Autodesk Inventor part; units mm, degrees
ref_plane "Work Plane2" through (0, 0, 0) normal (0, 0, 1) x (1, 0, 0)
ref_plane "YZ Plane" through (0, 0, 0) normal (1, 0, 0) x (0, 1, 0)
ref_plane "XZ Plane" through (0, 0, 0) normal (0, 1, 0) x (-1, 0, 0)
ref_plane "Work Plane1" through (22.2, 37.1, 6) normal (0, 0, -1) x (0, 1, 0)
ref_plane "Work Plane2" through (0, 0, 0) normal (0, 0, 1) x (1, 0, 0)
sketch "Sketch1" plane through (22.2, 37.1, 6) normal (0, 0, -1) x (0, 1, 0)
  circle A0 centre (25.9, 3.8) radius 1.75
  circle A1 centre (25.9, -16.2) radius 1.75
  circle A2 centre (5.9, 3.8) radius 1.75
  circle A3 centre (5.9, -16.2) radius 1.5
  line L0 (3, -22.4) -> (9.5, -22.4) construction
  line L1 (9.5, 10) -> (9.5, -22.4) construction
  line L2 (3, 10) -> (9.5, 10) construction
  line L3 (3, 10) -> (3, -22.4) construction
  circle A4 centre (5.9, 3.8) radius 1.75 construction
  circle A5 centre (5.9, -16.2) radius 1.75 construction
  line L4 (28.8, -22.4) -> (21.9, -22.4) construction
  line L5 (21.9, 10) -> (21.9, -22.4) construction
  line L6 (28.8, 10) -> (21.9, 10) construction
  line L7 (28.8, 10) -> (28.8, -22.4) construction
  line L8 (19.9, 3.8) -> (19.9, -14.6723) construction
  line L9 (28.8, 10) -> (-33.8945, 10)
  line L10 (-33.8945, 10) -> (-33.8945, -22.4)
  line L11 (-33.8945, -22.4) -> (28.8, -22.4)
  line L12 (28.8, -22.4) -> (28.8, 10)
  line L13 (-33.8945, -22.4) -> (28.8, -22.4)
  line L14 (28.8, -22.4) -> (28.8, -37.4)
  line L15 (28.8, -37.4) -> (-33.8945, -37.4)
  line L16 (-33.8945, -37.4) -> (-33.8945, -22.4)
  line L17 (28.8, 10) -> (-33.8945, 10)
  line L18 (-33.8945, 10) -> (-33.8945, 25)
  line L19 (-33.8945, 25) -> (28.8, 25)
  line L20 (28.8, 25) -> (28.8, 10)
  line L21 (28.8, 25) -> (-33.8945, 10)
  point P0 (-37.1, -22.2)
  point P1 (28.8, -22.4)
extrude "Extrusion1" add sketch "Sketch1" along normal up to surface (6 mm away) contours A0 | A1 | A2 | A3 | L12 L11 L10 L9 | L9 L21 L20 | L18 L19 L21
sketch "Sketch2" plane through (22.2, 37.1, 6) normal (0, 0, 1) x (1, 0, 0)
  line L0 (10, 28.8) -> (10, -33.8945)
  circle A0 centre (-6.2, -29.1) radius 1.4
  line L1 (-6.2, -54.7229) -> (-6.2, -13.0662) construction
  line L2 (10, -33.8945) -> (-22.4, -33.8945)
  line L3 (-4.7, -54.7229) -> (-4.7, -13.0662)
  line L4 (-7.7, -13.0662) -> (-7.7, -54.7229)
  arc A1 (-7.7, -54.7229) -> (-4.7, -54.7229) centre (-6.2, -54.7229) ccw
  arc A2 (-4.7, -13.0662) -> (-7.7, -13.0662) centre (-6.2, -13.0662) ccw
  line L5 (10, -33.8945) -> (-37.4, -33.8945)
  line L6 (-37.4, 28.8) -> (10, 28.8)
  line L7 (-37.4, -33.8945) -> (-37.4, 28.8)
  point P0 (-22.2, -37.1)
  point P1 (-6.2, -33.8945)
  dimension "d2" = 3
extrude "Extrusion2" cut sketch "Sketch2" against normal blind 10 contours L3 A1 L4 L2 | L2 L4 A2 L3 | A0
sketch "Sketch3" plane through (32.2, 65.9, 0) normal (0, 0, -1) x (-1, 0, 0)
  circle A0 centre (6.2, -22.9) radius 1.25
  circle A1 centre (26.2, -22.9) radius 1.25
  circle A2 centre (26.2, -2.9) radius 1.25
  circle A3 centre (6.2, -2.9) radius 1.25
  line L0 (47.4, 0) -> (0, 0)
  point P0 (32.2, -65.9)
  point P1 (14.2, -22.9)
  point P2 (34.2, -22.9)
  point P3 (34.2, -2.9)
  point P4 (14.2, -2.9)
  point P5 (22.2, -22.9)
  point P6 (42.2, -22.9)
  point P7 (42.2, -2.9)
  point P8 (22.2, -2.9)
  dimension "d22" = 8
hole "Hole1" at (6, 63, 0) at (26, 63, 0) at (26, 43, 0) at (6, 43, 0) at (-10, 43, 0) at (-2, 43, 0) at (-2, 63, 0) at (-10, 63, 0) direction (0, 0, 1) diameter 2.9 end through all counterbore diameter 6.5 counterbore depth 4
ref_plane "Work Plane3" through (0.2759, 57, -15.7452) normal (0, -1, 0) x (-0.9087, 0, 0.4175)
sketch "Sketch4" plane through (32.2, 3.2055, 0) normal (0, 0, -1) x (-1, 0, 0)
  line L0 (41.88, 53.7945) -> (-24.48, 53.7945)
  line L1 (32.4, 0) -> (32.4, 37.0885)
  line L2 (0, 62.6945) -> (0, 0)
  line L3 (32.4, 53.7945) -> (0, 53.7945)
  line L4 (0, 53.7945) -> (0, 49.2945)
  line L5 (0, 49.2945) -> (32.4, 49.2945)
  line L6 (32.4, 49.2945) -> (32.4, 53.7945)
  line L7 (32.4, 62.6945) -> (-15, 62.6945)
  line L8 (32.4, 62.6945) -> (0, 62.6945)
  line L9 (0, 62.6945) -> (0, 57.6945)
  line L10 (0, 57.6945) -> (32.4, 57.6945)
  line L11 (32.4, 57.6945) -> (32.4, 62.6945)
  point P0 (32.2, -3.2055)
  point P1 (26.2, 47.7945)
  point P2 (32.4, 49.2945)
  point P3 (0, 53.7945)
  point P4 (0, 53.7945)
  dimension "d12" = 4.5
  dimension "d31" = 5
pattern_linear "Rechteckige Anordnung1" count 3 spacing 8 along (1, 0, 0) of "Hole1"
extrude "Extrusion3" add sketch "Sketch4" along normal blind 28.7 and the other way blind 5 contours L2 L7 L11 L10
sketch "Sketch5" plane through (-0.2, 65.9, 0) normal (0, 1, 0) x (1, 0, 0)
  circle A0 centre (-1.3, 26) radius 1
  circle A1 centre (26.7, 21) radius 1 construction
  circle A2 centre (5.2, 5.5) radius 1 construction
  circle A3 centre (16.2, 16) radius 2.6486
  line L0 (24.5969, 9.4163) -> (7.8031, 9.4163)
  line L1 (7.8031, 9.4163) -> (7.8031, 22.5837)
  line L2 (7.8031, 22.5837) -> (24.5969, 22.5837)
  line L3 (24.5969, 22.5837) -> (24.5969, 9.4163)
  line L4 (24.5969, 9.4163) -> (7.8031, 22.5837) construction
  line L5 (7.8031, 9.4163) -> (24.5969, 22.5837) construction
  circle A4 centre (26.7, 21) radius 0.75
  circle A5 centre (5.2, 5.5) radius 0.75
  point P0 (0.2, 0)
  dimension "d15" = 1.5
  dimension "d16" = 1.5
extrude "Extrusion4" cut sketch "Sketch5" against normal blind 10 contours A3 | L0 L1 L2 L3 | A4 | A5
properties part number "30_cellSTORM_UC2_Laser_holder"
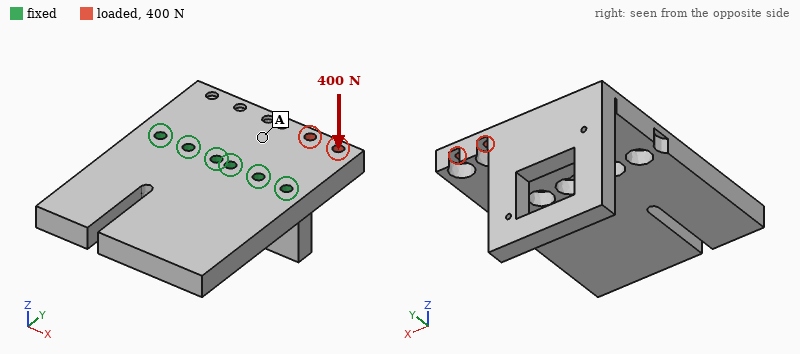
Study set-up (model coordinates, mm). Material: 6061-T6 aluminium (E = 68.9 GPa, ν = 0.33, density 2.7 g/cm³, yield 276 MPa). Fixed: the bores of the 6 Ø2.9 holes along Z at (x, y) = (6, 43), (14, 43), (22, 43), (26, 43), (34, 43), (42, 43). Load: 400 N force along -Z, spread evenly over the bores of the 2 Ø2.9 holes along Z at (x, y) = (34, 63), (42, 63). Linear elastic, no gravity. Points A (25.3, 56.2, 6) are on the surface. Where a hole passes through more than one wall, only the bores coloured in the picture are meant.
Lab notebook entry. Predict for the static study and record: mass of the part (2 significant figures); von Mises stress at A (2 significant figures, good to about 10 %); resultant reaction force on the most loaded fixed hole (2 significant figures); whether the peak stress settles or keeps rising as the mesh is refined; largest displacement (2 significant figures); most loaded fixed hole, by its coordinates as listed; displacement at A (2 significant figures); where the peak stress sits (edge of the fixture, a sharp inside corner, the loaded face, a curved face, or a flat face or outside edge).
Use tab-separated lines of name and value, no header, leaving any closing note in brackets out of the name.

mass of the part	53 g
von Mises stress at A	16 MPa
resultant reaction force on the most loaded fixed hole	180 N
whether the peak stress settles or keeps rising as the mesh is refined	keeps rising
largest displacement	0.14 mm
most loaded fixed hole, by its coordinates as listed	(42, 43)
displacement at A	0.040 mm
where the peak stress sits	edge of the fixture
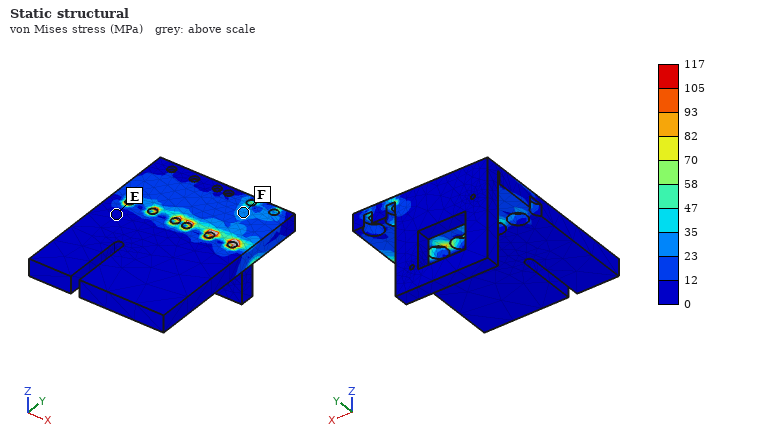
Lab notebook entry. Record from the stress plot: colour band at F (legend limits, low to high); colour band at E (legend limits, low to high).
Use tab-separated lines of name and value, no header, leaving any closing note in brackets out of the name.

colour band at F	23 to 35 MPa
colour band at E	0 to 12 MPa
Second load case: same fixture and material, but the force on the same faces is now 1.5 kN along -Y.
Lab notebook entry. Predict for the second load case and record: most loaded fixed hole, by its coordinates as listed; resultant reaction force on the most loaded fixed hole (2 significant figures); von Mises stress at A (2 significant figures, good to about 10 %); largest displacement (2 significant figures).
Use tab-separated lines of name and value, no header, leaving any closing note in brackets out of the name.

most loaded fixed hole, by its coordinates as listed	(42, 43)
resultant reaction force on the most loaded fixed hole	740 N
von Mises stress at A	12 MPa
largest displacement	22 µm
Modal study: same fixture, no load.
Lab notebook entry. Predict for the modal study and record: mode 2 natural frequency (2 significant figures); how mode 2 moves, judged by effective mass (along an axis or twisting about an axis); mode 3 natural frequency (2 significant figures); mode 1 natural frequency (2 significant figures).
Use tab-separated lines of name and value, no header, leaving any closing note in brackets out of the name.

mode 2 natural frequency	2600 Hz
how mode 2 moves, judged by effective mass	along Z
mode 3 natural frequency	3700 Hz
mode 1 natural frequency	1600 Hz
